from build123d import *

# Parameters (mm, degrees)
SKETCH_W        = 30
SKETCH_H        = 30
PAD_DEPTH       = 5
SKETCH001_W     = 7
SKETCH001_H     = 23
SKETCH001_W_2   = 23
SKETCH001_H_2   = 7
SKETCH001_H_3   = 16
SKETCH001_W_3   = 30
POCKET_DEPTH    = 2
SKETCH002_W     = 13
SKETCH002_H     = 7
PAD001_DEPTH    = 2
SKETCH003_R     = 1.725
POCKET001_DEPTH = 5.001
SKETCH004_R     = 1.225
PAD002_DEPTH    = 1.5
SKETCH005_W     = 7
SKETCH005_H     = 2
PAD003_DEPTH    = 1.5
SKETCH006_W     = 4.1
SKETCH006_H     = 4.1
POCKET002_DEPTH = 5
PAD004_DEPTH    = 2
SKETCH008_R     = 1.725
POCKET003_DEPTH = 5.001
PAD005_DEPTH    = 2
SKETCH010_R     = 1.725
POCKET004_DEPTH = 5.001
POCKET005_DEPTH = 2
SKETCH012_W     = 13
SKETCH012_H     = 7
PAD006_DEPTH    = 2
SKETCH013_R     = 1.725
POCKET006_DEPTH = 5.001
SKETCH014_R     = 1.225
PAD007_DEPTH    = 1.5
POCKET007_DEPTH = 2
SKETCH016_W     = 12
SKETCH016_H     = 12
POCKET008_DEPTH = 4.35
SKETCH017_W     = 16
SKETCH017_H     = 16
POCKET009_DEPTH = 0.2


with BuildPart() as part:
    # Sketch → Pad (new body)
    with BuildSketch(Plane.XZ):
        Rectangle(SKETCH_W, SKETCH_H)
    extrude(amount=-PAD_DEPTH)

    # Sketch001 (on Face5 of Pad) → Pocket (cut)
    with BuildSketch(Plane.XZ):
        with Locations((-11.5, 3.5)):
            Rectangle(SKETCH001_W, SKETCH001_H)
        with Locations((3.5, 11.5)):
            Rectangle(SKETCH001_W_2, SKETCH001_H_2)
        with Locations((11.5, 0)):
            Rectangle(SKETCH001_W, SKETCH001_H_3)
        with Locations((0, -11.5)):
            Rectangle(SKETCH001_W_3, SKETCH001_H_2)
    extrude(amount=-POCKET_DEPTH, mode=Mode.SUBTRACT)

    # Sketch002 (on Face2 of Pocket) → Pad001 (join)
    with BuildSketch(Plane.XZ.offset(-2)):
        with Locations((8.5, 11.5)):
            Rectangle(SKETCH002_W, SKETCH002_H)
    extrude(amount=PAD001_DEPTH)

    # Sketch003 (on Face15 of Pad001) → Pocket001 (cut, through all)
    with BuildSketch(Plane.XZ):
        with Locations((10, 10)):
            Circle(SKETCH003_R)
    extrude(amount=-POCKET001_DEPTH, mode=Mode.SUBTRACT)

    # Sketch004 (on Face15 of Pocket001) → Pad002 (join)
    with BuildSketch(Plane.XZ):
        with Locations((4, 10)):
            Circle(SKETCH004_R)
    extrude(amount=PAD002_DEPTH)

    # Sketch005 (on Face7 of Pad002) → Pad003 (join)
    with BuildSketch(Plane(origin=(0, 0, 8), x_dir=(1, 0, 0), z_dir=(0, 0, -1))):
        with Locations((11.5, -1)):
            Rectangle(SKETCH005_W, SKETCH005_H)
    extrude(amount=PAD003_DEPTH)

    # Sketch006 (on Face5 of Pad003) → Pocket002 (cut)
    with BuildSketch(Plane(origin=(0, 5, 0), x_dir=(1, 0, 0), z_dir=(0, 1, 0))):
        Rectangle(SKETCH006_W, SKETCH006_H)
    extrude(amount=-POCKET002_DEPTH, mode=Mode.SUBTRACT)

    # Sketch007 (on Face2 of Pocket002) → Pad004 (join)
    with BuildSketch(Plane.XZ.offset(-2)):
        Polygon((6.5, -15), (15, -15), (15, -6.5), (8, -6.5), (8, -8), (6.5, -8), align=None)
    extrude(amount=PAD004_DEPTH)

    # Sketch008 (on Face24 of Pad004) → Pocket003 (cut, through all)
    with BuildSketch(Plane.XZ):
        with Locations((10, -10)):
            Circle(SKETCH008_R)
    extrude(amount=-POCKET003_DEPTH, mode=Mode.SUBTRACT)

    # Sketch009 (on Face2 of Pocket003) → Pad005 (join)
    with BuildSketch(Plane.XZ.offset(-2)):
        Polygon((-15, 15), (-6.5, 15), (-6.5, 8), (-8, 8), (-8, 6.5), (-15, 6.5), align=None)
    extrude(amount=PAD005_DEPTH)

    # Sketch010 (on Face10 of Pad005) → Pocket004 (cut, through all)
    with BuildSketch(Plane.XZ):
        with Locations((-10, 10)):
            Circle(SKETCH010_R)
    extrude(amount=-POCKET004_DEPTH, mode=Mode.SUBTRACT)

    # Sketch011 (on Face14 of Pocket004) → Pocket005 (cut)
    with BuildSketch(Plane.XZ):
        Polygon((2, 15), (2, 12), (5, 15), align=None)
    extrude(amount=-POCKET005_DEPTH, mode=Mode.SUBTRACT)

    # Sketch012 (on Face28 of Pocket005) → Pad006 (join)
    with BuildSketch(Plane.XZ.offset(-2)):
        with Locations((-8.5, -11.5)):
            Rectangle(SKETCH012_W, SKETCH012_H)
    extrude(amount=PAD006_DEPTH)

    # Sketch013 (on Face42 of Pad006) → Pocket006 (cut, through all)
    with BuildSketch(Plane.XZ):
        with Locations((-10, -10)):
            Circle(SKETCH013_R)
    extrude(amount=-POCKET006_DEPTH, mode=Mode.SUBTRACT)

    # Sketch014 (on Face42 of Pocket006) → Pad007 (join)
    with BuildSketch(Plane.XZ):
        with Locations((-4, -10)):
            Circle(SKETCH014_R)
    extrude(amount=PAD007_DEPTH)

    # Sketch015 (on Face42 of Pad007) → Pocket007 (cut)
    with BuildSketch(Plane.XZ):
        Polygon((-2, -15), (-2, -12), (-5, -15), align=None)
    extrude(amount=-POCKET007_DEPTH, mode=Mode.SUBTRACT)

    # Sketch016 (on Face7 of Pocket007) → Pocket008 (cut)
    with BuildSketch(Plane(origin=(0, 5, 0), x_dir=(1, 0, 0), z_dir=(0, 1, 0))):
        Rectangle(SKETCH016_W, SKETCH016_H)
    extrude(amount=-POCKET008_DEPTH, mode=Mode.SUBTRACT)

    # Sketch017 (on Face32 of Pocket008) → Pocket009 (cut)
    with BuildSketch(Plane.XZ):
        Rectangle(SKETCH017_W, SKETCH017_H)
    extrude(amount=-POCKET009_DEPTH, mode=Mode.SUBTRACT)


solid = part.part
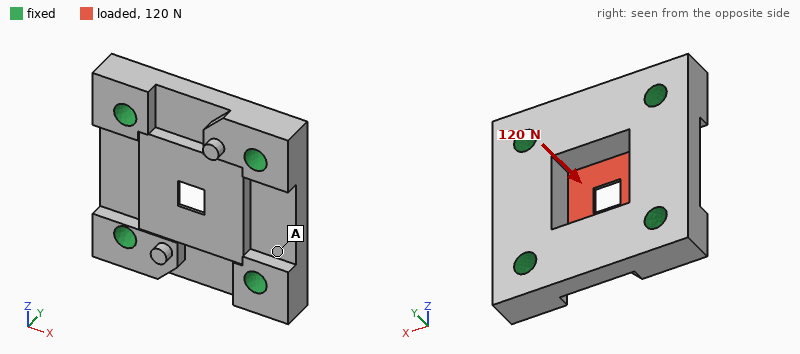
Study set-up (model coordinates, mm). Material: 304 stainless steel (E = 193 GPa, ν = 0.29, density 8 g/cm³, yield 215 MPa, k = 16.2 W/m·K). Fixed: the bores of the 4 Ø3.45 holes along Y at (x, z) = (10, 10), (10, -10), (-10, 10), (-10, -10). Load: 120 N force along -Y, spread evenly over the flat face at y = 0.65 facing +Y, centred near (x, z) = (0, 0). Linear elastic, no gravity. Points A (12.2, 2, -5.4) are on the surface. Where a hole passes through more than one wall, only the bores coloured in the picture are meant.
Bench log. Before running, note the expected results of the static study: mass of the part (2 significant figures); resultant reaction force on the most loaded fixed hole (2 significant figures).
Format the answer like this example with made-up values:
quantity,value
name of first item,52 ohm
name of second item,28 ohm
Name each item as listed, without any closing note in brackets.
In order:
quantity,value
mass of the part,24 g
resultant reaction force on the most loaded fixed hole,33 N
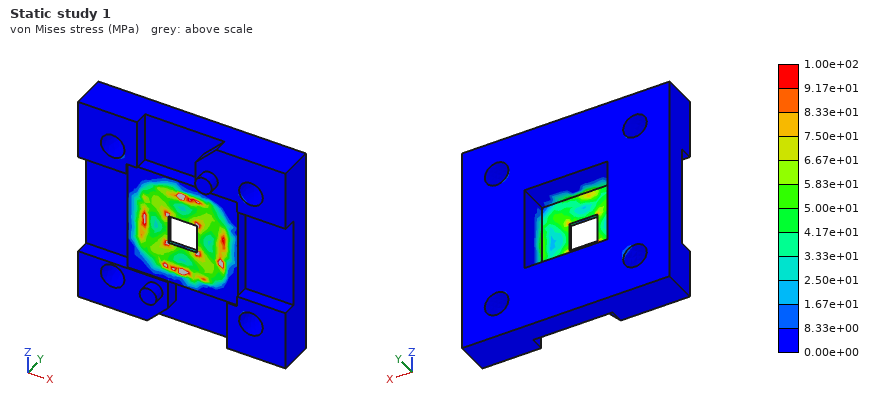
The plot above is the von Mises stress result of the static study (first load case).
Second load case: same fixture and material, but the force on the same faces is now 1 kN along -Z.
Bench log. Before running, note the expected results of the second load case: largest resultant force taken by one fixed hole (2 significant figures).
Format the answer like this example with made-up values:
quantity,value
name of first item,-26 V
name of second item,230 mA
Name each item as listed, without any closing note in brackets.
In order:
quantity,value
largest resultant force taken by one fixed hole,290 N
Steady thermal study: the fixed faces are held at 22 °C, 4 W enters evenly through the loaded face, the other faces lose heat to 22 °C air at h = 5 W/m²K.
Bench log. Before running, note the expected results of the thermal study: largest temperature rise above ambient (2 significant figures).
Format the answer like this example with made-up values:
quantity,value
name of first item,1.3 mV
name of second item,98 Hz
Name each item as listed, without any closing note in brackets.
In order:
quantity,value
largest temperature rise above ambient,46 K
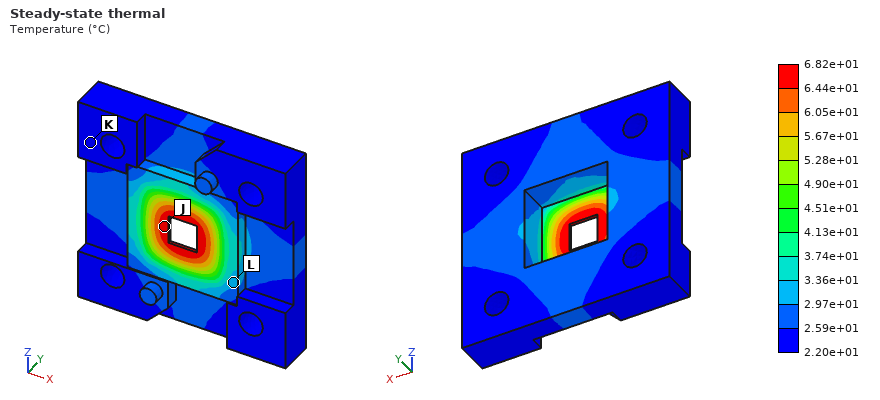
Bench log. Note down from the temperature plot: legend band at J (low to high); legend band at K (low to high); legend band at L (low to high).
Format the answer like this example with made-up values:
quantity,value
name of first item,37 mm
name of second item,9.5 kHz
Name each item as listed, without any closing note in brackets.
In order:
quantity,value
legend band at J,6.44e+01 to 6.82e+01 °C
legend band at K,2.20e+01 to 2.59e+01 °C
legend band at L,2.97e+01 to 3.36e+01 °C
